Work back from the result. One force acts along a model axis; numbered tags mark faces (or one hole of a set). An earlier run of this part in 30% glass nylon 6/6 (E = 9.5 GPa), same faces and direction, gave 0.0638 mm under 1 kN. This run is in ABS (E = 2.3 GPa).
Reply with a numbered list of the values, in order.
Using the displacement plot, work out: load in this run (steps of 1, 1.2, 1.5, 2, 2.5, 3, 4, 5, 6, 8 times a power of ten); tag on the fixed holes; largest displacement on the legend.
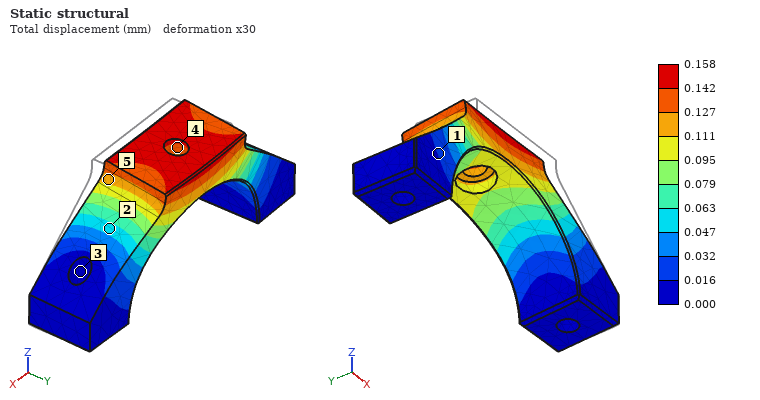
1. 600 N
2. 3
3. 0.158 mm
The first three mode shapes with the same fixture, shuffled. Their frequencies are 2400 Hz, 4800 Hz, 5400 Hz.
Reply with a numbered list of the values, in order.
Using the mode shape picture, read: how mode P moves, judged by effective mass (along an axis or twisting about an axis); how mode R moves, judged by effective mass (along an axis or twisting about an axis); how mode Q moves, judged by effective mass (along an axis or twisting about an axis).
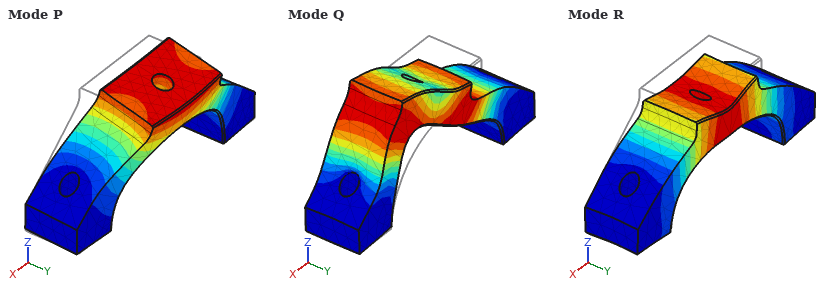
1. along Y
2. along Z
3. along X
